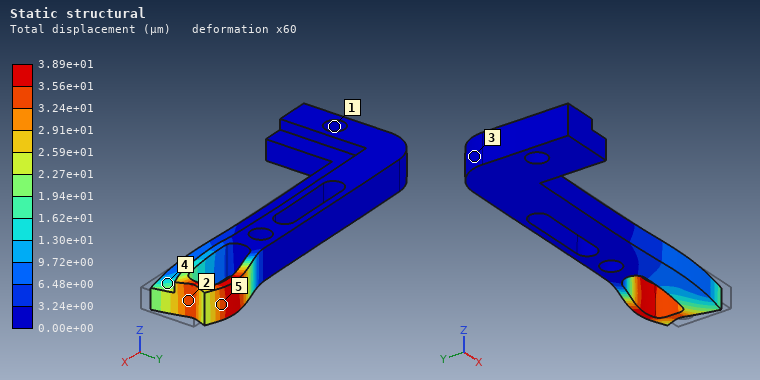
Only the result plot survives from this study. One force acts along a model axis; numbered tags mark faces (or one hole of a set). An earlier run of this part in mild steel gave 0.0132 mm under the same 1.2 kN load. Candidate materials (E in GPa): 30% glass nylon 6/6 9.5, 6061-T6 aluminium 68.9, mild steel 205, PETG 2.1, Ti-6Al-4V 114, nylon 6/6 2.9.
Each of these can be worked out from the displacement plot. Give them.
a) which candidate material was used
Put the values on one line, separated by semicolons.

6061-T6 aluminium
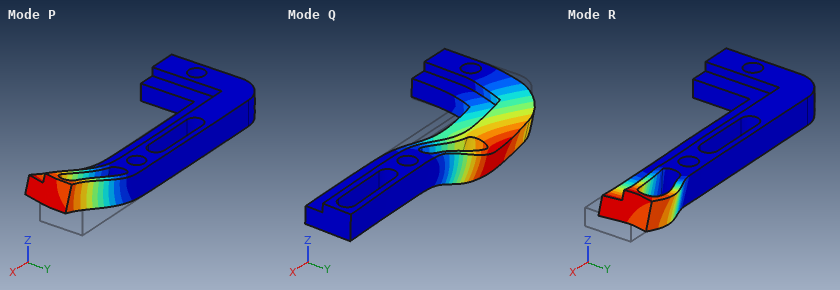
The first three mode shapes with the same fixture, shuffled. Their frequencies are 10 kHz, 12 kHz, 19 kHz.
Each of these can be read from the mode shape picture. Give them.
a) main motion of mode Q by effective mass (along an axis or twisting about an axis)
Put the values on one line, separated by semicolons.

along Z
